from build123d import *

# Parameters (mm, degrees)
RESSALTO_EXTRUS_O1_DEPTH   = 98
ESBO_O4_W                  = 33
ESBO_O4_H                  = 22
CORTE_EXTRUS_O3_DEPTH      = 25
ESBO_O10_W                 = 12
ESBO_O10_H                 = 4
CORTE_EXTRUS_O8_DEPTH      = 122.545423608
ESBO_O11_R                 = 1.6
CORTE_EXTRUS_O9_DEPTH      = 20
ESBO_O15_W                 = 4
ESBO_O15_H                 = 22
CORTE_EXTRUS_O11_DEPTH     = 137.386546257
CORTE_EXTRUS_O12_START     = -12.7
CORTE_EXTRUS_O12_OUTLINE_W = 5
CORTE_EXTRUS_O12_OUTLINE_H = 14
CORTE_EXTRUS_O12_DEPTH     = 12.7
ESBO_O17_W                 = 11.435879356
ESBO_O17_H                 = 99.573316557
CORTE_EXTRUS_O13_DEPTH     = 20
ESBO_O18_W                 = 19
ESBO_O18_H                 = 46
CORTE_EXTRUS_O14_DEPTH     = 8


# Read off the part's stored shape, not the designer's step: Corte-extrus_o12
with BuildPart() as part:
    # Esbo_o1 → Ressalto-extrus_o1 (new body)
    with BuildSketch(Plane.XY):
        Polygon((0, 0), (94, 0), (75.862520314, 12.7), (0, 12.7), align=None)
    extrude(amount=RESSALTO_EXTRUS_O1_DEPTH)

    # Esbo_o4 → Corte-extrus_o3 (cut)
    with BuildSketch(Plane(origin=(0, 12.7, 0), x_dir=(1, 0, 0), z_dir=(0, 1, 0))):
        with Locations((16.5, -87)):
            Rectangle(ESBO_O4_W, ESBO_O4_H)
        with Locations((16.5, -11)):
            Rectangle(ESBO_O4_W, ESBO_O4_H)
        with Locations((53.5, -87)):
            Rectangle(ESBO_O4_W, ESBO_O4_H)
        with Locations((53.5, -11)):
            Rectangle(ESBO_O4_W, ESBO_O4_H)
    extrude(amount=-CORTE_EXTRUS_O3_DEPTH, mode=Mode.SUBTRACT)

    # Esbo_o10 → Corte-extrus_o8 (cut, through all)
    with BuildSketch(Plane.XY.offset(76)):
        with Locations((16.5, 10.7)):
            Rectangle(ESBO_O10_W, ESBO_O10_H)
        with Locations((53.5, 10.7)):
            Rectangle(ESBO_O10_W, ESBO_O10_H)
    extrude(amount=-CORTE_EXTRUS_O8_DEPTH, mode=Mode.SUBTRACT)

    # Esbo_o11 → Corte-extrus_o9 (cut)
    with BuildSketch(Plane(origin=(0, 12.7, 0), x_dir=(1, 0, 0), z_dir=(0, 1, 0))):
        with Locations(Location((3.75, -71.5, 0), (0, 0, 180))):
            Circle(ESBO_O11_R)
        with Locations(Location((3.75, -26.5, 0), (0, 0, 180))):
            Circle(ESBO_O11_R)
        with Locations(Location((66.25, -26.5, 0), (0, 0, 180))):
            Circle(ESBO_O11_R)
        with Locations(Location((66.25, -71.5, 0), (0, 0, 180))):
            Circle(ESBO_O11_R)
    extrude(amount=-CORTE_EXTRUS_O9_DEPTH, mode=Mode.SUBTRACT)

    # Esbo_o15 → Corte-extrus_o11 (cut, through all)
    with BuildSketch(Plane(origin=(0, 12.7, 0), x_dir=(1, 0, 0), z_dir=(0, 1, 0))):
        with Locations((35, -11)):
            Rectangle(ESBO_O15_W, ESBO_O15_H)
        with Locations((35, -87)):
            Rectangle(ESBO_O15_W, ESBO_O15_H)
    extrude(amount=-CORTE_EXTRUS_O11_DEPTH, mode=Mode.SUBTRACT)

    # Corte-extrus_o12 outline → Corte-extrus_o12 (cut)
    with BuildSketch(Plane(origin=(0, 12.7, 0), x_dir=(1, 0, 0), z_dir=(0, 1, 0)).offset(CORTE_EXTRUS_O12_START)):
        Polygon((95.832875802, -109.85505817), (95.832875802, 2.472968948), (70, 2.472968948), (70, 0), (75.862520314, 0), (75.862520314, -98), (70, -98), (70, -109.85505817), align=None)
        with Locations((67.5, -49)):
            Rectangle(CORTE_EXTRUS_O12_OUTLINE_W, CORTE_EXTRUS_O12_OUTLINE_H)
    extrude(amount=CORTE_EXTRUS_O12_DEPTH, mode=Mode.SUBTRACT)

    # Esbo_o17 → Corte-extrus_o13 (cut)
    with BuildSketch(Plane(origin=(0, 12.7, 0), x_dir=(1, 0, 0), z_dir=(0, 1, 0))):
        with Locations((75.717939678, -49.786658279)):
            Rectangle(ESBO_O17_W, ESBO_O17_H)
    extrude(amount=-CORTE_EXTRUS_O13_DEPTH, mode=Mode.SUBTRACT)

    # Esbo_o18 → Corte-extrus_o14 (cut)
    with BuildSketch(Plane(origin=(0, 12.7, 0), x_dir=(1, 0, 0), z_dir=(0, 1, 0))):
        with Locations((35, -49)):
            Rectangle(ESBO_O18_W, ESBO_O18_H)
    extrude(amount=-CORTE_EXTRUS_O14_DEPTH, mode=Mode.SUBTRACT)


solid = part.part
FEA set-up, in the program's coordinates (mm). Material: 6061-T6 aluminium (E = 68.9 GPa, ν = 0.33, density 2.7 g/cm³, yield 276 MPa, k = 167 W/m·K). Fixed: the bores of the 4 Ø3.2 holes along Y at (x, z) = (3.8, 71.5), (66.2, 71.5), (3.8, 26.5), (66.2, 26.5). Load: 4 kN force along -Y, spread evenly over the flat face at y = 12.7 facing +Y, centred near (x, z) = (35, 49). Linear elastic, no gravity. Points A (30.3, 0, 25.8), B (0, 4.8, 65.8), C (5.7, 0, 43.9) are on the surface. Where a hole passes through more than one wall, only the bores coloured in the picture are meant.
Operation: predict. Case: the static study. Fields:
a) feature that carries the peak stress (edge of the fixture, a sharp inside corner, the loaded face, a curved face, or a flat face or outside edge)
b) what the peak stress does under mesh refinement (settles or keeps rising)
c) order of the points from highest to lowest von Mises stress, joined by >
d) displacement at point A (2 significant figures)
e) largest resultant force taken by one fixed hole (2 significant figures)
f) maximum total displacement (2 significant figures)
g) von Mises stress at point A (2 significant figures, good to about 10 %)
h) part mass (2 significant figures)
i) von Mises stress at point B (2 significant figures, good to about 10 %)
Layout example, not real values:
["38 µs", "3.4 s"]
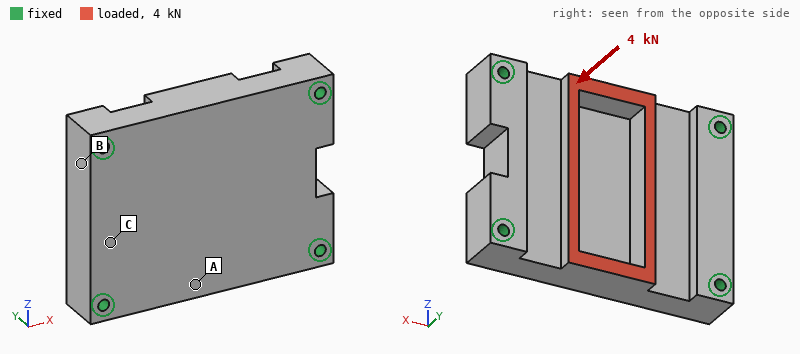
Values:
["edge of the fixture", "keeps rising", "A > B > C", "28 µm", "1.3 kN", "31 µm", "29 MPa", "93 g", "16 MPa"]
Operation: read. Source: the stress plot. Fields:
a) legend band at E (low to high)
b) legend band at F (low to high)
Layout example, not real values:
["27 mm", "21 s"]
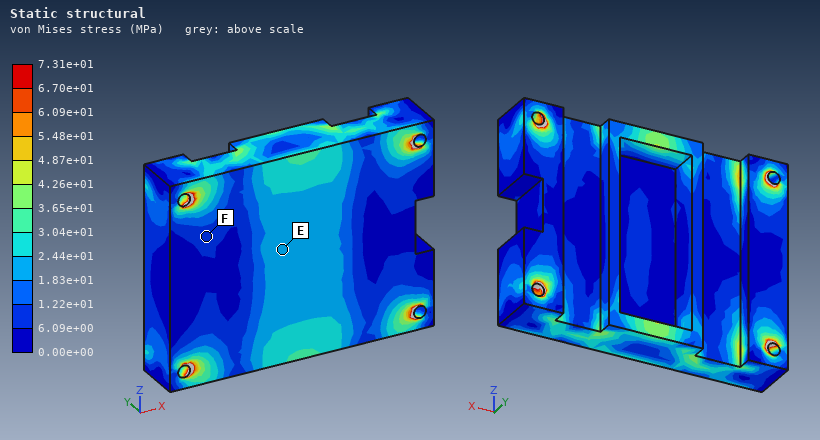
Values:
["1.83e+01 to 2.44e+01 MPa", "6.09e+00 to 1.22e+01 MPa"]
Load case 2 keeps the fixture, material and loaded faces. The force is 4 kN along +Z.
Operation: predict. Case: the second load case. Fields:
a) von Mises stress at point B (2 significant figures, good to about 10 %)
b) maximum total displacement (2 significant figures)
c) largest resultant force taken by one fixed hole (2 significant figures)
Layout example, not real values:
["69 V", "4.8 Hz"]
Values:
["5.1 MPa", "34 µm", "1.2 kN"]
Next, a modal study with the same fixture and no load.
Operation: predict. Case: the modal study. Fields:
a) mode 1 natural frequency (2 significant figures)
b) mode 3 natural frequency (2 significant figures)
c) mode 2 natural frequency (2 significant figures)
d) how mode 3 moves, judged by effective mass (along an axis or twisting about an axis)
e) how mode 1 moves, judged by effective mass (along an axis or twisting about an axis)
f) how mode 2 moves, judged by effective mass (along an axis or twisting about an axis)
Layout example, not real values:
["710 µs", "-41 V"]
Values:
["9500 Hz", "17 kHz", "14 kHz", "twisting about Z", "along Y", "twisting about X"]
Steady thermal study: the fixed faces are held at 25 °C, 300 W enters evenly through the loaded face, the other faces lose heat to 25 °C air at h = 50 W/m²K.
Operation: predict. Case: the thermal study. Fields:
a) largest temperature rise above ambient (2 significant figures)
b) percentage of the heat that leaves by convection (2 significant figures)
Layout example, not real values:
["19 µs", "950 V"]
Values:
["83 K", "6.4 %"]
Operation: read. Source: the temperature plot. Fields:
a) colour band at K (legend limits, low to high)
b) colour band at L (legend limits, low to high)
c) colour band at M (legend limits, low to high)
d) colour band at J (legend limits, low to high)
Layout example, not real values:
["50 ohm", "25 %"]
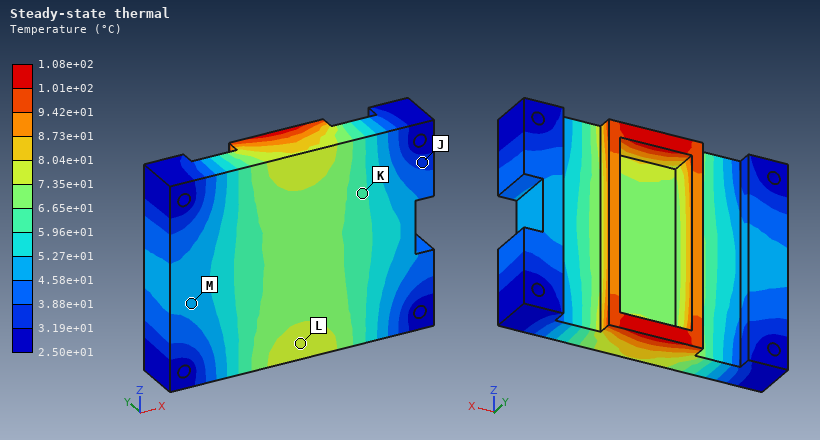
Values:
["5.96e+01 to 6.65e+01 °C", "7.35e+01 to 8.04e+01 °C", "4.58e+01 to 5.27e+01 °C", "3.19e+01 to 3.88e+01 °C"]
